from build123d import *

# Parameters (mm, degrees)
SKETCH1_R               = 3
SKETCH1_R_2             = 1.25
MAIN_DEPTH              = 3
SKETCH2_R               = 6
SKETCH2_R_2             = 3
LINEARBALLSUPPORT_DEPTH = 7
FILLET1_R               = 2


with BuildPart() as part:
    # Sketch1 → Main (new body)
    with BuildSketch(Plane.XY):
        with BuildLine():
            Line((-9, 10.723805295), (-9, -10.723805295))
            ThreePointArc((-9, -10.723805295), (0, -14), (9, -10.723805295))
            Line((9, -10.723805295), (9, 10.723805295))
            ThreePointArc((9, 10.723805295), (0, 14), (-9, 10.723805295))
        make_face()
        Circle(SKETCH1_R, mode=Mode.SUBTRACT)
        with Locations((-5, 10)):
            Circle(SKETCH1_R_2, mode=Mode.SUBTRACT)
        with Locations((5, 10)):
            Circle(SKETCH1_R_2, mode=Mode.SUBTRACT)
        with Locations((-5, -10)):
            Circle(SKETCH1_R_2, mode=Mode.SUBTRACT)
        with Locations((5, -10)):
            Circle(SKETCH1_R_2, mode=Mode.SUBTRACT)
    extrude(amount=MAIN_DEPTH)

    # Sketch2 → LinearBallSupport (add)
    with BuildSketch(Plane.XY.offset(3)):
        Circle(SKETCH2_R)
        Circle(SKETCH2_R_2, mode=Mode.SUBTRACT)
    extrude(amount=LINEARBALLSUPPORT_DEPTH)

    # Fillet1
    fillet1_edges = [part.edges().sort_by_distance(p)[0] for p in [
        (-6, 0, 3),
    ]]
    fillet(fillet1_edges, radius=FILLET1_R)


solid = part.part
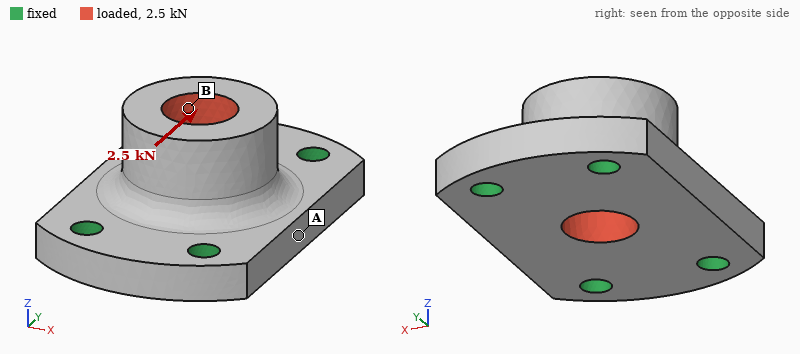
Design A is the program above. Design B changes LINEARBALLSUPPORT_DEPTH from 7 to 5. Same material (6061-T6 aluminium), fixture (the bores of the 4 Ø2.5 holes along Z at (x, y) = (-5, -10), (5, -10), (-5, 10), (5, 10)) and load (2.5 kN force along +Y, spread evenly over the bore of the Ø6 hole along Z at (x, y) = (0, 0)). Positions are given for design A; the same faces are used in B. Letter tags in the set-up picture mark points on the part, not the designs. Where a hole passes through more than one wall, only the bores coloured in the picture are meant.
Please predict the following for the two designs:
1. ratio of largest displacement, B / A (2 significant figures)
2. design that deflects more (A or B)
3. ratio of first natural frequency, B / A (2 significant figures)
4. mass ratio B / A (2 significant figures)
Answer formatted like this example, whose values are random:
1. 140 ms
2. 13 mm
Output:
1. 0.66
2. A
3. 1.2
4. 0.91
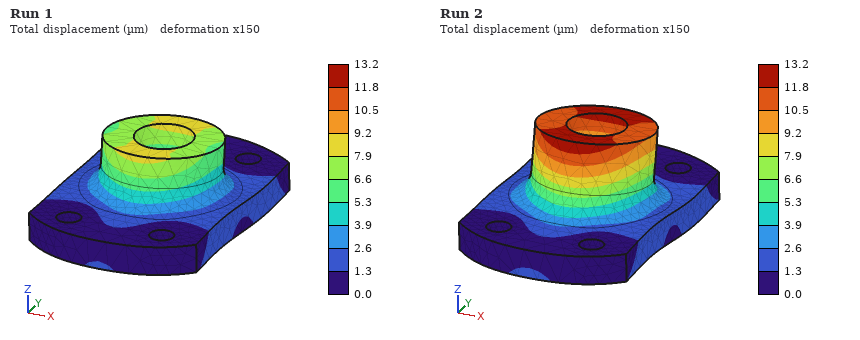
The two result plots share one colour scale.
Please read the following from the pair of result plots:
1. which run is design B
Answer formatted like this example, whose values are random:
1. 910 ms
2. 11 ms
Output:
1. Run 1
